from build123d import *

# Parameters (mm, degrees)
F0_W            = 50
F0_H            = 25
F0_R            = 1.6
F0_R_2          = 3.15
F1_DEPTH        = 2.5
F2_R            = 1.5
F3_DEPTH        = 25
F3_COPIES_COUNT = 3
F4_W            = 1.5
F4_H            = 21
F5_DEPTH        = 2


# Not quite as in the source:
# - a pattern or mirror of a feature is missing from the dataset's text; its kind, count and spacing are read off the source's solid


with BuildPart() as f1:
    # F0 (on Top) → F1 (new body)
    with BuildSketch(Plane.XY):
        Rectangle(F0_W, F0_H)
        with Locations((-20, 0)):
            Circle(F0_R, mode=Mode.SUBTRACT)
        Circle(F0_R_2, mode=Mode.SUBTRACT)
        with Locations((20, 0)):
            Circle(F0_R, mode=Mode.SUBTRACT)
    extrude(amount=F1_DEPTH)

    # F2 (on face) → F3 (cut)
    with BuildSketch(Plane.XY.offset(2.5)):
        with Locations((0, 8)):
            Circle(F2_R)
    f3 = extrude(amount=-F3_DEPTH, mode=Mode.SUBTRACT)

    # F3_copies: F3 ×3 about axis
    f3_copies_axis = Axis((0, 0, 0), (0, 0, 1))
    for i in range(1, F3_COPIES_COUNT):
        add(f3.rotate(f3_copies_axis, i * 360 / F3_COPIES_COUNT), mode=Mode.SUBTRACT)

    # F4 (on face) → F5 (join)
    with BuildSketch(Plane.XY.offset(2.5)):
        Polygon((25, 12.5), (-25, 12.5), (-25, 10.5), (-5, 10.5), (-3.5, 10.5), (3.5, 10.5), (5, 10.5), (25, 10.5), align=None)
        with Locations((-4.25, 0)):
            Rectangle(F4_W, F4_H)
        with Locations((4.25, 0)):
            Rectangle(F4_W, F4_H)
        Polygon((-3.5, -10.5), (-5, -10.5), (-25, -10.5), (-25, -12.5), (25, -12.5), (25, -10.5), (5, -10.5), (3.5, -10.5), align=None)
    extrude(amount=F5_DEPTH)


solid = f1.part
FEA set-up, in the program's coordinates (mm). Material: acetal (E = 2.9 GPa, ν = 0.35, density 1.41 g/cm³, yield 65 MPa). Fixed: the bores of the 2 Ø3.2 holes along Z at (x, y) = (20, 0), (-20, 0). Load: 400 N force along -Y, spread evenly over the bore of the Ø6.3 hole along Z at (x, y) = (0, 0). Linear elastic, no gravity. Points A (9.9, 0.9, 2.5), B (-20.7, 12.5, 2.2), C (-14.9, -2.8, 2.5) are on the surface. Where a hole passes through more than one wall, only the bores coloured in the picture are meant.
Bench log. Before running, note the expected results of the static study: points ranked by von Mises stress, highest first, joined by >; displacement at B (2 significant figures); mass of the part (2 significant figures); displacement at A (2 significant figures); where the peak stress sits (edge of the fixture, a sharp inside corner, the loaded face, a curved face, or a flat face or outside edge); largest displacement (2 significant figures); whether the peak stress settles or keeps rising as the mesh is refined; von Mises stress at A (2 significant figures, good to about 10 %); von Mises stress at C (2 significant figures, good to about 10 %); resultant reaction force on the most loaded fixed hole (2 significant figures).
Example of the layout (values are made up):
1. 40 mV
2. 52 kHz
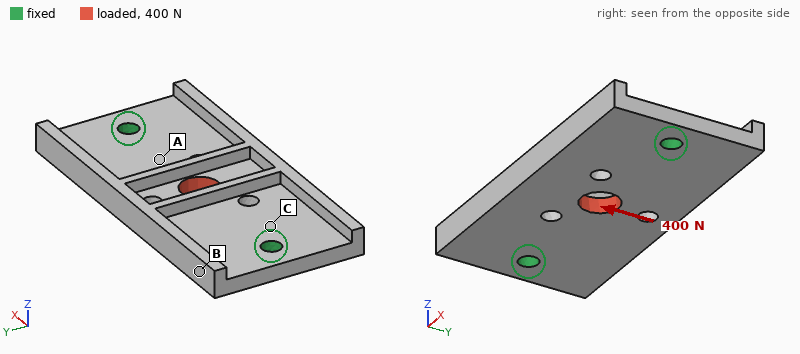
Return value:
1. C > A > B
2. 0.039 mm
3. 4.9 g
4. 0.070 mm
5. edge of the fixture
6. 0.14 mm
7. keeps rising
8. 7.7 MPa
9. 9.7 MPa
10. 200 N
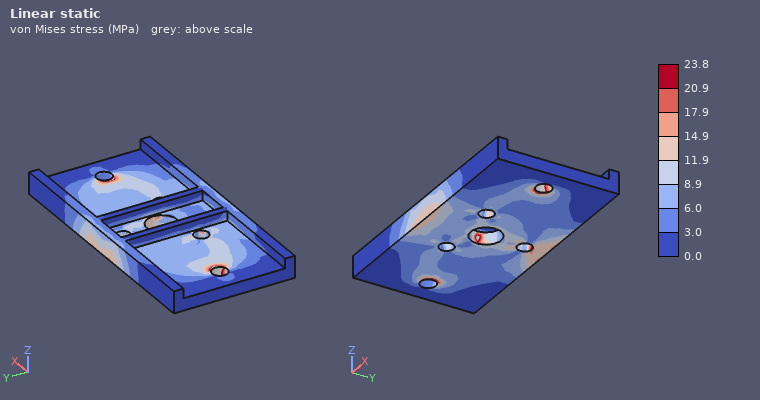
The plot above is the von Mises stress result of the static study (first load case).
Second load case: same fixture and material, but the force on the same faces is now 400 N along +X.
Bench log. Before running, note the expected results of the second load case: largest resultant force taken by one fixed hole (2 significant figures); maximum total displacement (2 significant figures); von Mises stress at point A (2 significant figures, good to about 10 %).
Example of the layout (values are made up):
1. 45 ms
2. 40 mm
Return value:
1. 200 N
2. 50 µm
3. 7.7 MPa
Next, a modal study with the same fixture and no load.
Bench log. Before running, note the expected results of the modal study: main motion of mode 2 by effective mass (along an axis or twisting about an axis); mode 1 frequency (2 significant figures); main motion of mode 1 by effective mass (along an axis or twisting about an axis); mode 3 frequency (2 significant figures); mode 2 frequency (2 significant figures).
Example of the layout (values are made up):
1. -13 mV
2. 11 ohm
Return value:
1. along Z
2. 1800 Hz
3. twisting about X
4. 3500 Hz
5. 2000 Hz
